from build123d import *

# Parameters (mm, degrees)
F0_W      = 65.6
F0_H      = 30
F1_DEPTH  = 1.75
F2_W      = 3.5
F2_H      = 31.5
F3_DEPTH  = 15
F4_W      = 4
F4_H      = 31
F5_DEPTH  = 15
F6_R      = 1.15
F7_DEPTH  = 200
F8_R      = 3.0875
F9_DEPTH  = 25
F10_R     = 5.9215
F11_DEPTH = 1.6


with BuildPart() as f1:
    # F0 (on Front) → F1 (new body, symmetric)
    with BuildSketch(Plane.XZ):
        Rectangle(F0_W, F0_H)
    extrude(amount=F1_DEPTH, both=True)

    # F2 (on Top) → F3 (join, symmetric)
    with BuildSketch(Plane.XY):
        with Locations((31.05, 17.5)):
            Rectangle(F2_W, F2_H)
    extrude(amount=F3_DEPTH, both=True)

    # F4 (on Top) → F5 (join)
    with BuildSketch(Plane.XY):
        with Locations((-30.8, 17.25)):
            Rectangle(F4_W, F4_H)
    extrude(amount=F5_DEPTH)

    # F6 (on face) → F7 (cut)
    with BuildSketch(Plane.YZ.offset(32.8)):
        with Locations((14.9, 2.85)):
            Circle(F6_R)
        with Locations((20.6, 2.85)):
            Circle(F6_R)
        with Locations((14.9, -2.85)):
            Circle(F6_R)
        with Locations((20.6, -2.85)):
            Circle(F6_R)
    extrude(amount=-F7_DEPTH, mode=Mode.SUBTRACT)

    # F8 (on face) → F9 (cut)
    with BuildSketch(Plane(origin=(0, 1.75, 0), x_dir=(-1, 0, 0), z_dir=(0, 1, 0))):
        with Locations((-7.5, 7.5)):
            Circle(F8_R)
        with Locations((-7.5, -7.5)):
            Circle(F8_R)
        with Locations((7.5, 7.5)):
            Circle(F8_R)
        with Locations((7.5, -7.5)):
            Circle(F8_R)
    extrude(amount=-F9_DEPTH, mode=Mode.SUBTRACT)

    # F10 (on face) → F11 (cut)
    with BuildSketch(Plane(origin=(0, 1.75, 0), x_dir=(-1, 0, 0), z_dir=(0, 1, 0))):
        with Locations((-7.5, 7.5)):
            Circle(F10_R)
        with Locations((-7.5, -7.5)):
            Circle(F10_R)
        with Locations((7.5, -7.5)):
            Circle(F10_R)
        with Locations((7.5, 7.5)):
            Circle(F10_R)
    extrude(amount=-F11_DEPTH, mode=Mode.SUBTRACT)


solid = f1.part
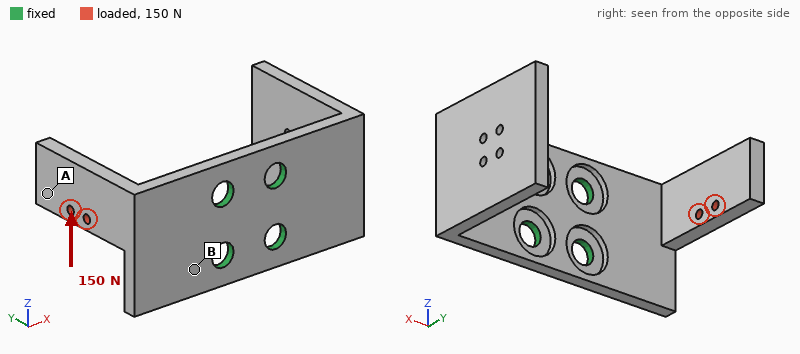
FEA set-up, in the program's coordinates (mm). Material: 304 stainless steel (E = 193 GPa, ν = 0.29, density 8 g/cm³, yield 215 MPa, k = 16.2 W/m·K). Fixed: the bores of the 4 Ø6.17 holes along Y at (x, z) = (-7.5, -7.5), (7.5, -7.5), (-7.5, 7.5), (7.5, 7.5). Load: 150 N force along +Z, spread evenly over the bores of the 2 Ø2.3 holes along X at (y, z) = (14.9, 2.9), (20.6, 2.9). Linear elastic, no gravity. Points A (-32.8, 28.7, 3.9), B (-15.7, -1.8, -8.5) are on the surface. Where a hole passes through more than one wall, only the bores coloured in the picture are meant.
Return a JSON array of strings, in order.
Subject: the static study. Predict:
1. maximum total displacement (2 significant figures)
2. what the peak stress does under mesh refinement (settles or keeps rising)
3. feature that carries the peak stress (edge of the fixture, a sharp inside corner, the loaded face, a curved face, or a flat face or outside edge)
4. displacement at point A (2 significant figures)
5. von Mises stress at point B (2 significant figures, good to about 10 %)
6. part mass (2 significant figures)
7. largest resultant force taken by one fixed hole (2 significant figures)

["73 µm", "keeps rising", "edge of the fixture", "59 µm", "18 MPa", "88 g", "290 N"]
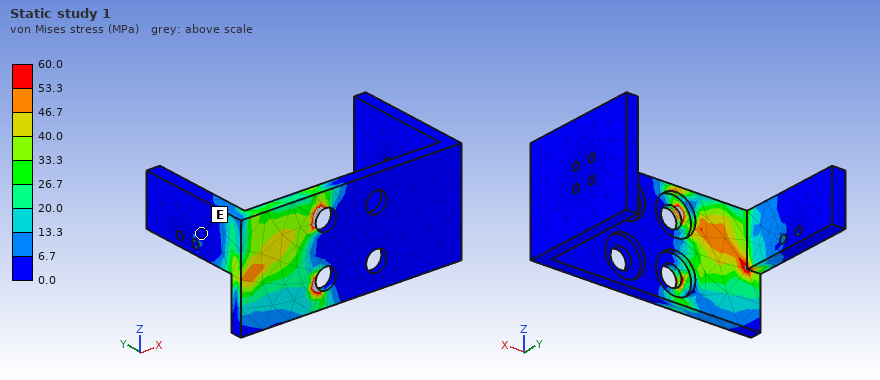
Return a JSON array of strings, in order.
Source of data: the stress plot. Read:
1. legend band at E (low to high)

["0.0 to 6.7 MPa"]
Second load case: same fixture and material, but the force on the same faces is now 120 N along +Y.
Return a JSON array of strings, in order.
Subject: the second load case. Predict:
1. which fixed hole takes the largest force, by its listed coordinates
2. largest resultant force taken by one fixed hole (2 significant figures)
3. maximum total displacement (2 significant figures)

["(-7.5, 7.5)", "130 N", "82 µm"]
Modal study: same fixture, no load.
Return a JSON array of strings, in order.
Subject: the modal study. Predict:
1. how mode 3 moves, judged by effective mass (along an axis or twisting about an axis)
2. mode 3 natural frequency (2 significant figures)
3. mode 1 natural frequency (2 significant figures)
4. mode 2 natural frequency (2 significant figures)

["along Z", "1900 Hz", "1000 Hz", "1300 Hz"]
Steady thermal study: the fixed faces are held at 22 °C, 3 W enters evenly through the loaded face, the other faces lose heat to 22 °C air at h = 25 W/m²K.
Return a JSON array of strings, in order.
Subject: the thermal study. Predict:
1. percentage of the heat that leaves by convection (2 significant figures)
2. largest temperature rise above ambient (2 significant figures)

["61 %", "63 K"]
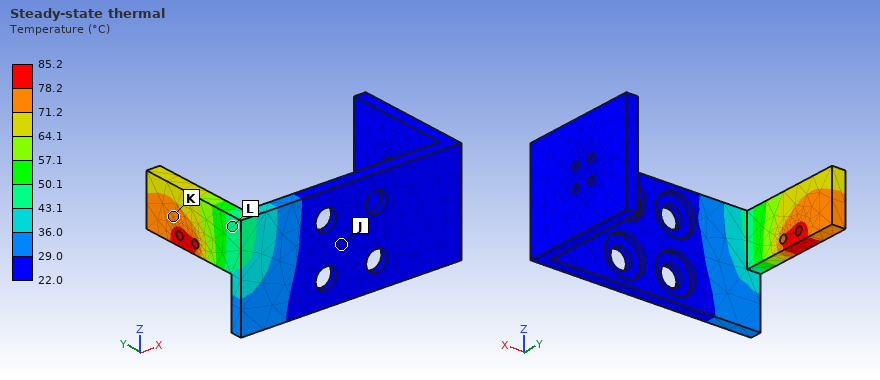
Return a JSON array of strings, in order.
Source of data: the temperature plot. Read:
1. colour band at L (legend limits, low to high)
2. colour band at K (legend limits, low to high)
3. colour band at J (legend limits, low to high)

["43.1 to 50.1 °C", "71.2 to 78.2 °C", "22.0 to 29.0 °C"]
